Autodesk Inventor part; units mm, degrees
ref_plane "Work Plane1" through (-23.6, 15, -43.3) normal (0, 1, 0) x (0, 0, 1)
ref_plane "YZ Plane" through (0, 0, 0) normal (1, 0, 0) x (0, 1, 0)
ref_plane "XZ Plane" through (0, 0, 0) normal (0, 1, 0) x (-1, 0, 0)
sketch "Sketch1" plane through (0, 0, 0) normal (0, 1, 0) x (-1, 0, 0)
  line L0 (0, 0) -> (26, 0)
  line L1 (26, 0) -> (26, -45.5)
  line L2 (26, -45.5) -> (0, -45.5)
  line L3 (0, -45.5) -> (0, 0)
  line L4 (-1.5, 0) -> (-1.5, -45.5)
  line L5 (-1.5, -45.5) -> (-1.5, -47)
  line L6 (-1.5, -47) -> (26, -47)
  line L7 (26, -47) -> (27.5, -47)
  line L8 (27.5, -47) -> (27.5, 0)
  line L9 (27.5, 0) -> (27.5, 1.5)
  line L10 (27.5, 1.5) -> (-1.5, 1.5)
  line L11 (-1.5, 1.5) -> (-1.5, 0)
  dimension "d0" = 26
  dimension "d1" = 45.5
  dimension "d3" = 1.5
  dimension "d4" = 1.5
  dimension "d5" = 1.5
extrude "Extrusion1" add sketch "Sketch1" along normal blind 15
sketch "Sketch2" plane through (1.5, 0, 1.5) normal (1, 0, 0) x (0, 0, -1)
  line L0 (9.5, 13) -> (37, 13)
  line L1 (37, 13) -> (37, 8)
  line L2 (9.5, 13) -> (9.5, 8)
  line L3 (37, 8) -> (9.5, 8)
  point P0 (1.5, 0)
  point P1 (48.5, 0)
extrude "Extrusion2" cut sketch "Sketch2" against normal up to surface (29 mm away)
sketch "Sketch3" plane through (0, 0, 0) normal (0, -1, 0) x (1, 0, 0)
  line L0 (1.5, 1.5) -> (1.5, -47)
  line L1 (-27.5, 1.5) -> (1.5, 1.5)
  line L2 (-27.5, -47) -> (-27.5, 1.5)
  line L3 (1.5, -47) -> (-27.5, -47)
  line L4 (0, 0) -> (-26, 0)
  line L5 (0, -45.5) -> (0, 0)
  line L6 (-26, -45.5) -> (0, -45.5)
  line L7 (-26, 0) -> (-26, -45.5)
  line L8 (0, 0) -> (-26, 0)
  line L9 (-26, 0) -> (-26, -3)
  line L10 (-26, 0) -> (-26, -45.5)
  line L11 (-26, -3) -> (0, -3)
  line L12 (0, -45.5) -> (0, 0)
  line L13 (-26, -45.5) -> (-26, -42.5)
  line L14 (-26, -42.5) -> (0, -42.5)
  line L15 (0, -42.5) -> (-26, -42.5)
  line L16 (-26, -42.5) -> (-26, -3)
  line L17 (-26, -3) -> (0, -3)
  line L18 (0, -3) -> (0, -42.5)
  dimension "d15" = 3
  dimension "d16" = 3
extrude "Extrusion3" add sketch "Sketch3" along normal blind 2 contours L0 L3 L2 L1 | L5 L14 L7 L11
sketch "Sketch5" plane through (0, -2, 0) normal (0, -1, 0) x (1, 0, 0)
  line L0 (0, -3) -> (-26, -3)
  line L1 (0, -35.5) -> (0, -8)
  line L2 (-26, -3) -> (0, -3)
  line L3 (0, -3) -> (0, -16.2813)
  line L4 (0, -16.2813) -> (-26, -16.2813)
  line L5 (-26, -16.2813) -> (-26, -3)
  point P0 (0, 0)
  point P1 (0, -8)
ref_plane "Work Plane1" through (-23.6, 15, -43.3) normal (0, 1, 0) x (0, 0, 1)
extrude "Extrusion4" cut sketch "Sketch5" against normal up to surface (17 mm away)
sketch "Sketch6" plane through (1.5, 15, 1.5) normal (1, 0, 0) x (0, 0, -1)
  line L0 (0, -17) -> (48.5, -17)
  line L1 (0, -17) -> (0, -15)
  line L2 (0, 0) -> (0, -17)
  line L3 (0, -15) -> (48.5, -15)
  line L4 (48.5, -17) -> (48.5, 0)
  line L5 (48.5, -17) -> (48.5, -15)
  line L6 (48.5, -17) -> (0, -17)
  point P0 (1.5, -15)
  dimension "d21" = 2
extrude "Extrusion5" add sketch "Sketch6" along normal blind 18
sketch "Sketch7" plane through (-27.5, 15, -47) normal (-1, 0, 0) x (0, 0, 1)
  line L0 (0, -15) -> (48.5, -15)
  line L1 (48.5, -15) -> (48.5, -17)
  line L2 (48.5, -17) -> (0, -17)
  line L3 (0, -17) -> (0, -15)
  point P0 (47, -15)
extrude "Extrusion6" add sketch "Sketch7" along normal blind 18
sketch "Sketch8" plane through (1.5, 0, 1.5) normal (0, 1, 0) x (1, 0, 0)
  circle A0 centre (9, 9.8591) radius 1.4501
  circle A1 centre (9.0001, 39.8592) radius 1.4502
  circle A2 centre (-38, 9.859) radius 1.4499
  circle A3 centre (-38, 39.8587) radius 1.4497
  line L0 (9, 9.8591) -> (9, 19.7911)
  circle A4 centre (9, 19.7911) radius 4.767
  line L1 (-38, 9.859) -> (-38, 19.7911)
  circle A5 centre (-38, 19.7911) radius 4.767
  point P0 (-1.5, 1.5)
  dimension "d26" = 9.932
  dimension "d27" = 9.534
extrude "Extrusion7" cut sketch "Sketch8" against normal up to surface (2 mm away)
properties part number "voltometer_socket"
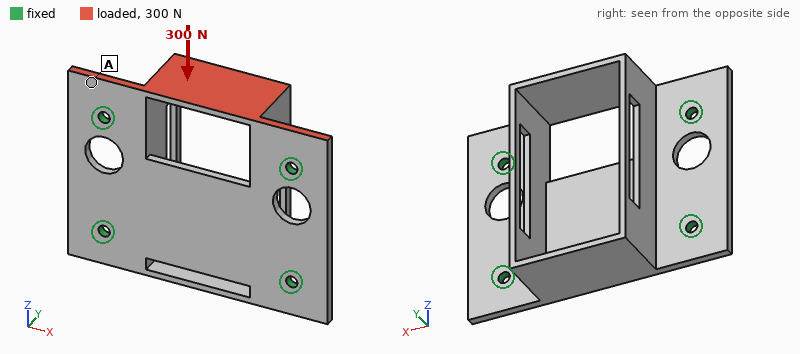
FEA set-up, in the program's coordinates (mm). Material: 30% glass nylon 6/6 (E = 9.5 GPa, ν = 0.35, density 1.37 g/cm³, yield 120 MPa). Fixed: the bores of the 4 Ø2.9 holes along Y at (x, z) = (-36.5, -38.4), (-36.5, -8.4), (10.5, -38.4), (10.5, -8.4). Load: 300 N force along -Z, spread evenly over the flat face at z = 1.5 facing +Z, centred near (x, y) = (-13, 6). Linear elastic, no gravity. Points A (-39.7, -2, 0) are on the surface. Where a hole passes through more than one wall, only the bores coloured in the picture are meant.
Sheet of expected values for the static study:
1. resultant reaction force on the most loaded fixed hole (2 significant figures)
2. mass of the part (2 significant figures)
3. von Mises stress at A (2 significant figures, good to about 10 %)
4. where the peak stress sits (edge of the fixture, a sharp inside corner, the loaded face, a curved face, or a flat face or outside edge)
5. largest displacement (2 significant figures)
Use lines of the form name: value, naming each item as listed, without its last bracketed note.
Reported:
resultant reaction force on the most loaded fixed hole: 86 N
mass of the part: 11 g
von Mises stress at A: 8.3 MPa
where the peak stress sits: the loaded face
largest displacement: 0.70 mm
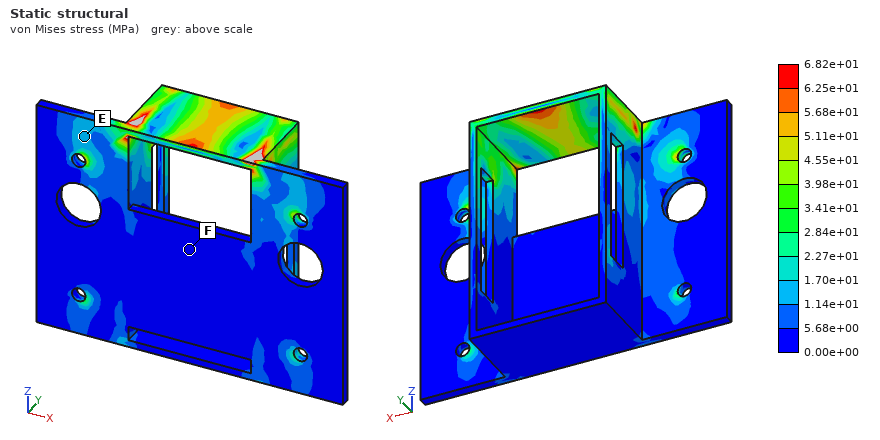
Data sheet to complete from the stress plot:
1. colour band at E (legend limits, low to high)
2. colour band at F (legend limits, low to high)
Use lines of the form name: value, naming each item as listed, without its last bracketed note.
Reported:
colour band at E: 1.14e+01 to 1.70e+01 MPa
colour band at F: 0.00e+00 to 5.68e+00 MPa
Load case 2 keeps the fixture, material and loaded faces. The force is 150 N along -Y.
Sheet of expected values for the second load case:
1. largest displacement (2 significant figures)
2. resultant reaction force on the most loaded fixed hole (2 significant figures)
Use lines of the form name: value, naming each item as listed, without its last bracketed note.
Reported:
largest displacement: 0.26 mm
resultant reaction force on the most loaded fixed hole: 100 N
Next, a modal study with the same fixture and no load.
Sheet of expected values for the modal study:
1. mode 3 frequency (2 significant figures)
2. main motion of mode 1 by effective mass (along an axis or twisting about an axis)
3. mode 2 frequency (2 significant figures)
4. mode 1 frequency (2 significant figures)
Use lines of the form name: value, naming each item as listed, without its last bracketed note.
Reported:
mode 3 frequency: 3000 Hz
main motion of mode 1 by effective mass: along Y
mode 2 frequency: 2600 Hz
mode 1 frequency: 2300 Hz
